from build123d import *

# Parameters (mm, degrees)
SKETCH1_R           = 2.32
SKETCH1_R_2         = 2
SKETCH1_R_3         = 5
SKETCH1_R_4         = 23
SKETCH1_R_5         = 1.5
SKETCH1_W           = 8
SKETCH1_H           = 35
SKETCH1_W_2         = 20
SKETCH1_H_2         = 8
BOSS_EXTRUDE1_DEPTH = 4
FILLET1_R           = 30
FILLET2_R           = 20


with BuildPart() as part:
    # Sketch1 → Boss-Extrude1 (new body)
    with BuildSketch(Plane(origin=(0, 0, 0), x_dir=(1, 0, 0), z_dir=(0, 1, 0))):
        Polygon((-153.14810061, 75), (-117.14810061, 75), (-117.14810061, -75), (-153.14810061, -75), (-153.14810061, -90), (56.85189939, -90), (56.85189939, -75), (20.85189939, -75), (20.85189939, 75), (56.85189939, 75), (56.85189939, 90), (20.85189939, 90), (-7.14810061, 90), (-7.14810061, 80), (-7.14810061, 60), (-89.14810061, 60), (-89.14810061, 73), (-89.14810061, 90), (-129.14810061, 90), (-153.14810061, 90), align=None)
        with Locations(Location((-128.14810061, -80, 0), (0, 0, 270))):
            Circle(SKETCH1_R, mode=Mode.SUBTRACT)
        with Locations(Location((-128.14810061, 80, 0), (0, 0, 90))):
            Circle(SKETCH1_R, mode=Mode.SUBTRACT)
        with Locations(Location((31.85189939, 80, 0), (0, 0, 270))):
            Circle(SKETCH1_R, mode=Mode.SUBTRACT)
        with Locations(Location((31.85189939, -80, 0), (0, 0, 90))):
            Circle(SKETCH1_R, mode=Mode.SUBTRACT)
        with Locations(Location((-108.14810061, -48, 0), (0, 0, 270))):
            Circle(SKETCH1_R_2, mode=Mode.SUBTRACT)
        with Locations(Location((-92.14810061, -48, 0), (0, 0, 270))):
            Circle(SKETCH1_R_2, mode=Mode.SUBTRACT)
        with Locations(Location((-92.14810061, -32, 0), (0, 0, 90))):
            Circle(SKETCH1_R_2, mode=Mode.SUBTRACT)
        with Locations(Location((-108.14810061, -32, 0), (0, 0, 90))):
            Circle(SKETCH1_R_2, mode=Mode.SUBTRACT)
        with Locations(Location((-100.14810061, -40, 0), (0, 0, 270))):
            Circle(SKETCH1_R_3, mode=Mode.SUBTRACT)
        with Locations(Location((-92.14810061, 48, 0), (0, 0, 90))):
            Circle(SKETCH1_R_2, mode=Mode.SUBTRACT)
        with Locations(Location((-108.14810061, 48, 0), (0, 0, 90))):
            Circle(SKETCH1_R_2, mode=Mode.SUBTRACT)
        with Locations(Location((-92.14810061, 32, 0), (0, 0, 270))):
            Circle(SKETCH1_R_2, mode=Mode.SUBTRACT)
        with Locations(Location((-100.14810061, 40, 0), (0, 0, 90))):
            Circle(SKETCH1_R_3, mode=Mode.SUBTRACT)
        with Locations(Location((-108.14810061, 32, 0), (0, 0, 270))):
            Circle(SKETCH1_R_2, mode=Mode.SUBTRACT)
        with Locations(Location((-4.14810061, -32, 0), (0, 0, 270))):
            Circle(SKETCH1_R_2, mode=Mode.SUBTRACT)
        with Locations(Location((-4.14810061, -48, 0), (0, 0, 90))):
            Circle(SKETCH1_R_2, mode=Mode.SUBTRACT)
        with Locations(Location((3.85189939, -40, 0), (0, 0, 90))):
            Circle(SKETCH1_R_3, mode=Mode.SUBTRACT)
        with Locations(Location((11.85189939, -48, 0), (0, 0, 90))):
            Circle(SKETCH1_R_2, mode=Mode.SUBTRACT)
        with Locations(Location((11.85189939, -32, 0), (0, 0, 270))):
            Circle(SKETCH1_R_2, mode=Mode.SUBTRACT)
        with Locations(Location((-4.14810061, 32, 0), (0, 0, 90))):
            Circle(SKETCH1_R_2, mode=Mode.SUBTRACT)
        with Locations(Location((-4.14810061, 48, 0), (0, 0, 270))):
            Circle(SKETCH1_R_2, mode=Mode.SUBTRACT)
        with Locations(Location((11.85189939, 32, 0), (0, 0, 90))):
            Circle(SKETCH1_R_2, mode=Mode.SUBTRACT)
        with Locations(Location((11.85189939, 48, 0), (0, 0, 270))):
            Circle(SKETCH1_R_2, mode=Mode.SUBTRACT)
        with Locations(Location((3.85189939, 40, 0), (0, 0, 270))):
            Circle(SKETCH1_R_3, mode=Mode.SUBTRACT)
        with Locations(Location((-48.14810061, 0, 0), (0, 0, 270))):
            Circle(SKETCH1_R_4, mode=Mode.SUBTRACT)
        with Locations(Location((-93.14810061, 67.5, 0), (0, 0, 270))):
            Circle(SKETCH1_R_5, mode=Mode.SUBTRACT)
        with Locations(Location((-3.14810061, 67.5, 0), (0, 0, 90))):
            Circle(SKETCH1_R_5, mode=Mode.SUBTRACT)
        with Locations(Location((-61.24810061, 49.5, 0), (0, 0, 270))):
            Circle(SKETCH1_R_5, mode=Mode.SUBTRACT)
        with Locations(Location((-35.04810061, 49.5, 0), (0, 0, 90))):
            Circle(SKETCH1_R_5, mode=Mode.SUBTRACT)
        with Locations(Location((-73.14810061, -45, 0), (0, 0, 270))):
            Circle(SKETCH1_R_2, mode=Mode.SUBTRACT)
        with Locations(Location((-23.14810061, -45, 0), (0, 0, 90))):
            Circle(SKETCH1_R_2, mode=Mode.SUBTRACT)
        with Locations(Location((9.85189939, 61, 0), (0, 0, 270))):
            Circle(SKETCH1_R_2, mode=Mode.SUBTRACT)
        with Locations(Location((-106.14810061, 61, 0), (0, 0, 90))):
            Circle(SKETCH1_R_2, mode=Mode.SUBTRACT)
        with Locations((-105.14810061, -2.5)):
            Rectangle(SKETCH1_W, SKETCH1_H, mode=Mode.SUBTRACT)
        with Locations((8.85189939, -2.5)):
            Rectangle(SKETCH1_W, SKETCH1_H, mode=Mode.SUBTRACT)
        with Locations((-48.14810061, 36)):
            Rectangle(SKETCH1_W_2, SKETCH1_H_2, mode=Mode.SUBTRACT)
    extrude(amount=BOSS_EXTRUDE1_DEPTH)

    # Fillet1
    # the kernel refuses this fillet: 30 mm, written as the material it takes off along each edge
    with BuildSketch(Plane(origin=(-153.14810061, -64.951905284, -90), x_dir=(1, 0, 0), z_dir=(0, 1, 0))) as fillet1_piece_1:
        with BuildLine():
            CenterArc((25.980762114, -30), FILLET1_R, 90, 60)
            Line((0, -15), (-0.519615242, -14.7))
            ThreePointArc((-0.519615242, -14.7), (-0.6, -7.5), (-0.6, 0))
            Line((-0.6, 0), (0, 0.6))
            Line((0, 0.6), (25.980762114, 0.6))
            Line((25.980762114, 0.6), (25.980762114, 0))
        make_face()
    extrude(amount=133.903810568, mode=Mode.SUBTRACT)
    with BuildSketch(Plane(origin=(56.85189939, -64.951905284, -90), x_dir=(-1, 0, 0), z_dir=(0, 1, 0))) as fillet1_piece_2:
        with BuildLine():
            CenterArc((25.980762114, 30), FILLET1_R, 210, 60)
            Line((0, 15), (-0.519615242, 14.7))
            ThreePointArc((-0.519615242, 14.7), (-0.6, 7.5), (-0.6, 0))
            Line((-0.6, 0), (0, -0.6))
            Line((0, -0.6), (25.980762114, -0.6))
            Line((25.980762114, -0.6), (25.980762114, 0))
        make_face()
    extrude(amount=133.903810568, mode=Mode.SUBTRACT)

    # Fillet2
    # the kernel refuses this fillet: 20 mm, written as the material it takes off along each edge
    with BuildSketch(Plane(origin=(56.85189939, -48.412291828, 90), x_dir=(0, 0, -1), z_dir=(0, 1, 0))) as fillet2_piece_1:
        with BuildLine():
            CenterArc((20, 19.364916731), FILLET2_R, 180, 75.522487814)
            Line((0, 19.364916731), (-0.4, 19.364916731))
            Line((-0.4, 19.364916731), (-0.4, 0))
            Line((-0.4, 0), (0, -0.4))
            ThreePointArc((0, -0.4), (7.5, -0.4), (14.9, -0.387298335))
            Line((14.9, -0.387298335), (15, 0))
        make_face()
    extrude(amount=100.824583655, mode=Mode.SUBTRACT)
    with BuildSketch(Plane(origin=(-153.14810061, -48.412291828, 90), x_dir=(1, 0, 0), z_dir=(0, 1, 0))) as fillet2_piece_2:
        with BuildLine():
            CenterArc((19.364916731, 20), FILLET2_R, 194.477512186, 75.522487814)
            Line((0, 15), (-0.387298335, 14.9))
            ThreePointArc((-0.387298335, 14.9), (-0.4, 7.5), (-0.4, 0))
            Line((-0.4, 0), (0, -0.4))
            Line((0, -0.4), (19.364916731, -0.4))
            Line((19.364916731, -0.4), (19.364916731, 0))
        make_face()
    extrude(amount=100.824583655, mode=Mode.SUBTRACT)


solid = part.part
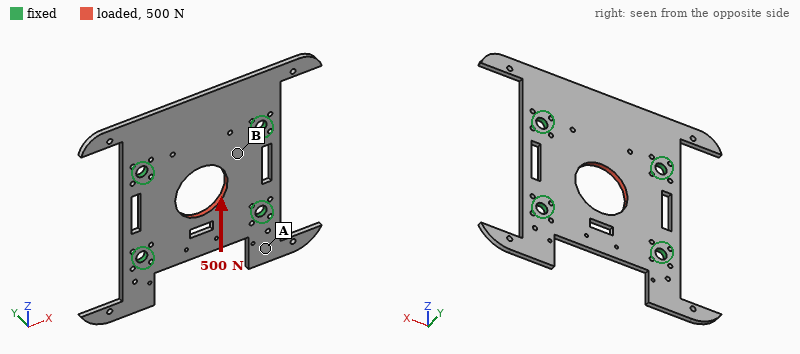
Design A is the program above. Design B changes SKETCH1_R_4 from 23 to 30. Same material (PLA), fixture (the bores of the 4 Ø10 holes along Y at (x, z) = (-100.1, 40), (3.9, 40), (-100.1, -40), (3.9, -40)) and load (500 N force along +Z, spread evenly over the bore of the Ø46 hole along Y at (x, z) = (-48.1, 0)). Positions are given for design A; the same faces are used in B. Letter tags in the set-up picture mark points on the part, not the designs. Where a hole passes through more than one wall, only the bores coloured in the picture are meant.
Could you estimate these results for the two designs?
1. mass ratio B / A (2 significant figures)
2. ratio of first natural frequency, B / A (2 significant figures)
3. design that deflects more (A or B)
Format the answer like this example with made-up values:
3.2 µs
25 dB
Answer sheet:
0.94
1.00
B
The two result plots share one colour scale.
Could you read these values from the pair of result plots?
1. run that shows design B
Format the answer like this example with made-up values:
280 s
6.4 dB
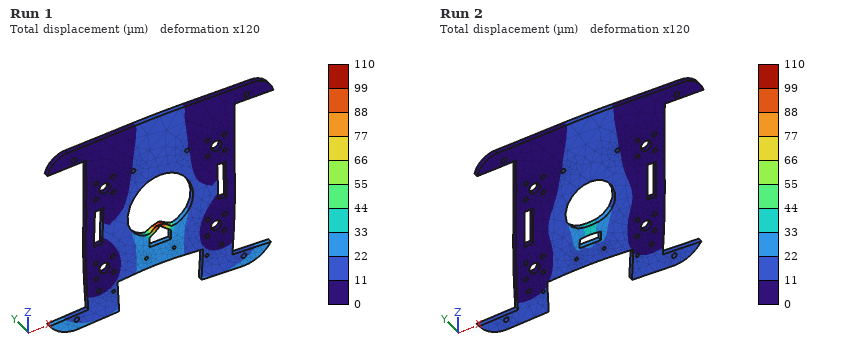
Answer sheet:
Run 1
